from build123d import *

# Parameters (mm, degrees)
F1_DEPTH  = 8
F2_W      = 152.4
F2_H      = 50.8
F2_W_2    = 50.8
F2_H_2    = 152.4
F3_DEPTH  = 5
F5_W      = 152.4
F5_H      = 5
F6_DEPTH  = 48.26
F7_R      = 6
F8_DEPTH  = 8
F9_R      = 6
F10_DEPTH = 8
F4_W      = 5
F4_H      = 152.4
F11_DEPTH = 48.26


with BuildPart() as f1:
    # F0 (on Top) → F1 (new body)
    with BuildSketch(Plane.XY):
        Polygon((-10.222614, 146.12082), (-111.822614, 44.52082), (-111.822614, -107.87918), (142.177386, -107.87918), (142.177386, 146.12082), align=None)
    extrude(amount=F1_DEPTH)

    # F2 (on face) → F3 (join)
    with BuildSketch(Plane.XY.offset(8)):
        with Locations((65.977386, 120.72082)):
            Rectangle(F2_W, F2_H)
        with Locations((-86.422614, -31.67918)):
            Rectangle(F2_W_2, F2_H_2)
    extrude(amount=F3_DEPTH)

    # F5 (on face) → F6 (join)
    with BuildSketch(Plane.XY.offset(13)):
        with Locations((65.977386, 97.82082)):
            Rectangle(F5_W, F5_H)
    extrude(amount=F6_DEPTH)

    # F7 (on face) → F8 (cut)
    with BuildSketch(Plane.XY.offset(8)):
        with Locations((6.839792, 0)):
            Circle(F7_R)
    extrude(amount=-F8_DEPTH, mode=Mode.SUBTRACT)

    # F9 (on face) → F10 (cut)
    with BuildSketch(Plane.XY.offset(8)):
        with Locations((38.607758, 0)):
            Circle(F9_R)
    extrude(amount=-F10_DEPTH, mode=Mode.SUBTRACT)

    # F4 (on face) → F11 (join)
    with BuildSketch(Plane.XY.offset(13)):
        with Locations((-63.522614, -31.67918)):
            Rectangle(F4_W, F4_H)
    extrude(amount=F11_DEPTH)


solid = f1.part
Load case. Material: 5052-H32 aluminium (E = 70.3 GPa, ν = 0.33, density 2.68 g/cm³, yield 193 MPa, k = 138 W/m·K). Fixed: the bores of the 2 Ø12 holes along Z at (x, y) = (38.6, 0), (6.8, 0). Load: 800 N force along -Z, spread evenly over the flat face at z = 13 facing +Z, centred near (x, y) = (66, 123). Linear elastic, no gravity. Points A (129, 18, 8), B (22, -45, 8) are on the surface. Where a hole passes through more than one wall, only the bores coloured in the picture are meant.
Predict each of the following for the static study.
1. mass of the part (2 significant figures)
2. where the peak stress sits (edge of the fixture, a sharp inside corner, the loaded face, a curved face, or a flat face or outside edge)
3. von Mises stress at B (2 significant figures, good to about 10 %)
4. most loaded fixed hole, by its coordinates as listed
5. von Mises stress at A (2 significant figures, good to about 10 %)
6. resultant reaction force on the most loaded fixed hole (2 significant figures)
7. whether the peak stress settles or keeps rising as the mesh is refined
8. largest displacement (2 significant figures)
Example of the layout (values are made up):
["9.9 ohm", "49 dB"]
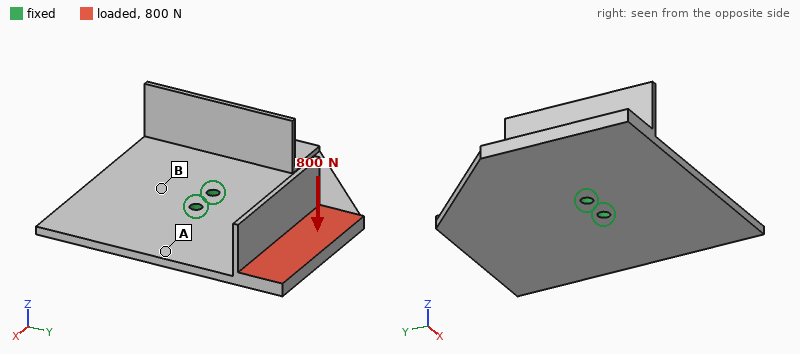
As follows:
["1.7 kg", "edge of the fixture", "8.5 MPa", "(38.6, 0)", "22 MPa", "980 N", "keeps rising", "1.5 mm"]
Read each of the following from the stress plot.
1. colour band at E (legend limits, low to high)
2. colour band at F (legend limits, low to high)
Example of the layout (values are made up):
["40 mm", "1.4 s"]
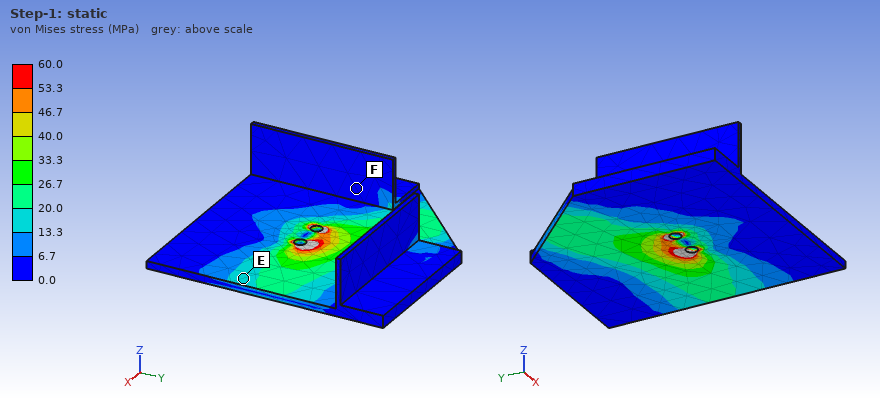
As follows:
["13.3 to 20.0 MPa", "0.0 to 6.7 MPa"]
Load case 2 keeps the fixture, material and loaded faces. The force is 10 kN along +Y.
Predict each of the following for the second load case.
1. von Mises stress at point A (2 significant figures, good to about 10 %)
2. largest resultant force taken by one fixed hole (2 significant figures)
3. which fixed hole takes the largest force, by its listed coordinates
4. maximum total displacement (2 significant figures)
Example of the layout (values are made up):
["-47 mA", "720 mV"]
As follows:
["31 MPa", "15 kN", "(38.6, 0)", "1.7 mm"]
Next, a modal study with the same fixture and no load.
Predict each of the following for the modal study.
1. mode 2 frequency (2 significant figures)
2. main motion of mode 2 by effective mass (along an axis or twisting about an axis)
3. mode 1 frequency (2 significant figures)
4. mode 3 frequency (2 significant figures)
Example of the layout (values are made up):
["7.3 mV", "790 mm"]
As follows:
["320 Hz", "along Z", "220 Hz", "390 Hz"]
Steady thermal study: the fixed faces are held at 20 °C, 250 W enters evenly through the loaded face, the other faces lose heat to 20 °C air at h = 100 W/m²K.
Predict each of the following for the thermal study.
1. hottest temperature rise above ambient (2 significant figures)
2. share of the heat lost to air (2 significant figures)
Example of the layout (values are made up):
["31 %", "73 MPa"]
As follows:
["62 K", "86 %"]
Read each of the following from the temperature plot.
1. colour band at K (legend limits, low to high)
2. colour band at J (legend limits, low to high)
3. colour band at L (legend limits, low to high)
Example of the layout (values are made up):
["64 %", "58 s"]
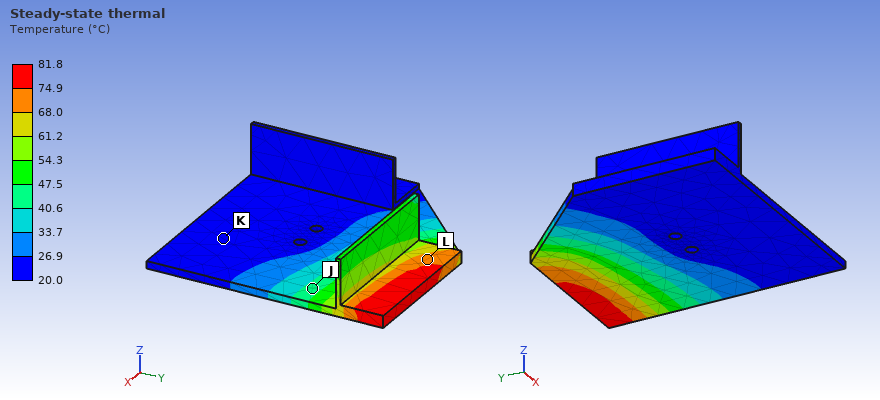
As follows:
["20.0 to 26.9 °C", "40.6 to 47.5 °C", "68.0 to 74.9 °C"]
